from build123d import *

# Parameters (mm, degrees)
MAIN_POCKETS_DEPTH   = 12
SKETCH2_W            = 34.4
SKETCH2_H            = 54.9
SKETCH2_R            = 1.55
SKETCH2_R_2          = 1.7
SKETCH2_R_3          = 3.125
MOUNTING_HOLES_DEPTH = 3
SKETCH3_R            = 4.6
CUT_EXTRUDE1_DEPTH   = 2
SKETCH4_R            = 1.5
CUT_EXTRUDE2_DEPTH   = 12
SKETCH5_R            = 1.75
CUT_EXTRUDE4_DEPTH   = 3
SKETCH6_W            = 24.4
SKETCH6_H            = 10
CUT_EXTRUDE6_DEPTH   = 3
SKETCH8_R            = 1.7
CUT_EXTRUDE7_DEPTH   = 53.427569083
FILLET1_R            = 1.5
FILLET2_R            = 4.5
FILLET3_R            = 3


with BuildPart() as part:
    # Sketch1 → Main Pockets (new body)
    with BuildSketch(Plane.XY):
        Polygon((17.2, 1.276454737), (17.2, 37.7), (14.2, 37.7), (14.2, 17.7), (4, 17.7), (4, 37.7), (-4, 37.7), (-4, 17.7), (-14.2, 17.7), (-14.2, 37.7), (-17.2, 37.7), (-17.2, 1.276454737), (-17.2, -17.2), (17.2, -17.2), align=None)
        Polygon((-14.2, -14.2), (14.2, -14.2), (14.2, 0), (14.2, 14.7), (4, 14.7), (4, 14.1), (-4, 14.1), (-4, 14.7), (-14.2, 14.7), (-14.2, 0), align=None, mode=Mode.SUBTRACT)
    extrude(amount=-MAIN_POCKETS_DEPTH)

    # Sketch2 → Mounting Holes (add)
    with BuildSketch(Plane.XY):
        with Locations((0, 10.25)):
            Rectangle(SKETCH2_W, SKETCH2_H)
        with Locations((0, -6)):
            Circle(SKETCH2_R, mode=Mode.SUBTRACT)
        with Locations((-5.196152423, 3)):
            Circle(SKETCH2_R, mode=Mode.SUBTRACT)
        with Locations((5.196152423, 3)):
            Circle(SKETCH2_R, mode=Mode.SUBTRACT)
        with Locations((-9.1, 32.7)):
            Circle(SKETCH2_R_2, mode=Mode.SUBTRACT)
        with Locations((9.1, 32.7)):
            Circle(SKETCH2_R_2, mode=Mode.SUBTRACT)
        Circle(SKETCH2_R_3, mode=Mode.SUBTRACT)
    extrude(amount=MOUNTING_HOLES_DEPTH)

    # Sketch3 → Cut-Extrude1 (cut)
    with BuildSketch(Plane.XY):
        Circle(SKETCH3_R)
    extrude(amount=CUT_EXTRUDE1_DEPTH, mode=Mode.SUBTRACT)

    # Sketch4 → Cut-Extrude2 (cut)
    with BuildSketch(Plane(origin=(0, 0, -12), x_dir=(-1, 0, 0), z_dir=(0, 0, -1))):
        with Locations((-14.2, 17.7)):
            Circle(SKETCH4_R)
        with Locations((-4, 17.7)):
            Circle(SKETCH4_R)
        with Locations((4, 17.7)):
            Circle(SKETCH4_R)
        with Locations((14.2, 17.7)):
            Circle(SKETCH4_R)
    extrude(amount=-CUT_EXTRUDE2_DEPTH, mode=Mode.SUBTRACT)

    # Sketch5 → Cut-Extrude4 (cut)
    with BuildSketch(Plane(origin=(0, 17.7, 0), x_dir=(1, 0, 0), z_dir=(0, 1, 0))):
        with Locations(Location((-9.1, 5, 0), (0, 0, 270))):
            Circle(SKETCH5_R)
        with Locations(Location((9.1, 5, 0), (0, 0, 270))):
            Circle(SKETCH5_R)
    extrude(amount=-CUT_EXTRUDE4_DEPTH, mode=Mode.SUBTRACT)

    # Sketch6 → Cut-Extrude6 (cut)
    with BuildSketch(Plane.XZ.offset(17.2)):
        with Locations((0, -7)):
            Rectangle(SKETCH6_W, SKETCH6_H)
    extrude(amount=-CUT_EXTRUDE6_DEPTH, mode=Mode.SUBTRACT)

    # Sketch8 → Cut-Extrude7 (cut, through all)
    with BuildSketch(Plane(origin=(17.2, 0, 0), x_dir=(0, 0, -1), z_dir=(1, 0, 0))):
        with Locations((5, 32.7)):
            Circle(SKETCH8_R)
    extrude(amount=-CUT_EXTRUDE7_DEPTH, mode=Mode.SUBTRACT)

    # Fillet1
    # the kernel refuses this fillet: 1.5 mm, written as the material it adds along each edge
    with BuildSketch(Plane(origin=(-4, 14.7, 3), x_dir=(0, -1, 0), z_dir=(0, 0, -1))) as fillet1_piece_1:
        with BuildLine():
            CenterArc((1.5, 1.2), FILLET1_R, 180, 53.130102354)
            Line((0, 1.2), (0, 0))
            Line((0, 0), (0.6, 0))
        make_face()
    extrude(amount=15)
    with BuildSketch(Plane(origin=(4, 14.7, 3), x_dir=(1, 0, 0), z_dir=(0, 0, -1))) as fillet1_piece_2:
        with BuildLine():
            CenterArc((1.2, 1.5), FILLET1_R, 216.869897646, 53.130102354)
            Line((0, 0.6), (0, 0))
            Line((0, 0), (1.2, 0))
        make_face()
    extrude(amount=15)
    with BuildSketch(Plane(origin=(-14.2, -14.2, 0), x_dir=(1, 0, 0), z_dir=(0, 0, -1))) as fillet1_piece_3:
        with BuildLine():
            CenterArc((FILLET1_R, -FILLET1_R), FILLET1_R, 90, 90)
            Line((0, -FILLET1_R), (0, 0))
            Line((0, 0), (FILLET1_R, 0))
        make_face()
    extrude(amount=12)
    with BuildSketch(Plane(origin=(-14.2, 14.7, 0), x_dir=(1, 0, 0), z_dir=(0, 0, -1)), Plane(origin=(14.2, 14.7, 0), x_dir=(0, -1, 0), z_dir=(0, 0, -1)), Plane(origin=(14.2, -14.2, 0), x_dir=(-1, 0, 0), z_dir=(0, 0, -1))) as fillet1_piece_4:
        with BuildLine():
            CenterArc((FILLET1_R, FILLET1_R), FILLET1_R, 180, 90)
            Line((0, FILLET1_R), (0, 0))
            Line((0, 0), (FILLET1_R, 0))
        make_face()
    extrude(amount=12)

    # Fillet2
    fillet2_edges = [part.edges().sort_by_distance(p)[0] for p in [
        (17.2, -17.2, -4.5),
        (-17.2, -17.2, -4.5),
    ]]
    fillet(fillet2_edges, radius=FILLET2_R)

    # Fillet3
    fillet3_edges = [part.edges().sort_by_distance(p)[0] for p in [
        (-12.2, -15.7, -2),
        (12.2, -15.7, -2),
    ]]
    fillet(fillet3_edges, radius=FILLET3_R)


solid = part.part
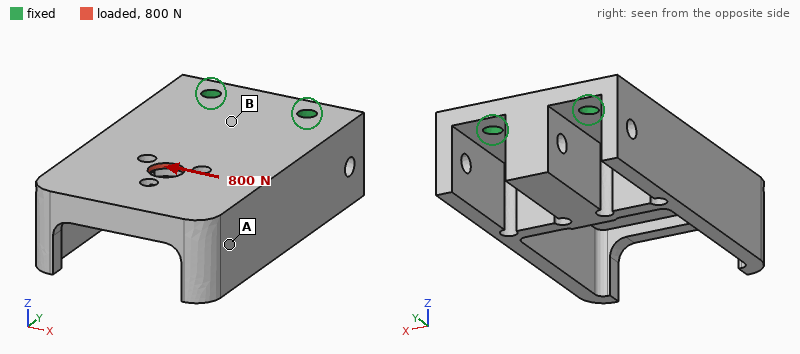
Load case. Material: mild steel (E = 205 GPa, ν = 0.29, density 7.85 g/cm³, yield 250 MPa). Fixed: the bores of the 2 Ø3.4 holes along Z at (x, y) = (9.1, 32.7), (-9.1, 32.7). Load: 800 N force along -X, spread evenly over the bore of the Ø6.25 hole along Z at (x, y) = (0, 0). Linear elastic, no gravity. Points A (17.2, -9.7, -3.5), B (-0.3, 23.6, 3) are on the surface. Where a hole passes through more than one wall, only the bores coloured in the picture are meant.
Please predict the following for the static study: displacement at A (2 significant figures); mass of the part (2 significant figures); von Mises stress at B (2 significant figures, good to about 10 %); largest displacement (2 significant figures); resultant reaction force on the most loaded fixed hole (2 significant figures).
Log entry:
14 µm
95 g
28 MPa
17 µm
1.3 kN
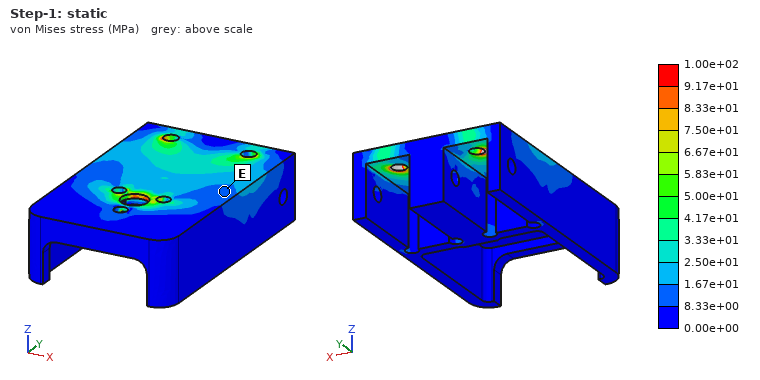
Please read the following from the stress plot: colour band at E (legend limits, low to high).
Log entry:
8.33e+00 to 1.67e+01 MPa
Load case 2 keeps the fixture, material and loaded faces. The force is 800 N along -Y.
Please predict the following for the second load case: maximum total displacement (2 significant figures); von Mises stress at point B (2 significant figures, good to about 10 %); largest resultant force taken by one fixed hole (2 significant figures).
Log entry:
11 µm
6.7 MPa
400 N
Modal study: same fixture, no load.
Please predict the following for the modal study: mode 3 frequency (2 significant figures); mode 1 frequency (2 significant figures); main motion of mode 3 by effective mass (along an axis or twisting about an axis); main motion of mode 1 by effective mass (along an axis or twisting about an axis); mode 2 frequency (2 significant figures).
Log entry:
5600 Hz
1600 Hz
along X
along Z
3100 Hz
